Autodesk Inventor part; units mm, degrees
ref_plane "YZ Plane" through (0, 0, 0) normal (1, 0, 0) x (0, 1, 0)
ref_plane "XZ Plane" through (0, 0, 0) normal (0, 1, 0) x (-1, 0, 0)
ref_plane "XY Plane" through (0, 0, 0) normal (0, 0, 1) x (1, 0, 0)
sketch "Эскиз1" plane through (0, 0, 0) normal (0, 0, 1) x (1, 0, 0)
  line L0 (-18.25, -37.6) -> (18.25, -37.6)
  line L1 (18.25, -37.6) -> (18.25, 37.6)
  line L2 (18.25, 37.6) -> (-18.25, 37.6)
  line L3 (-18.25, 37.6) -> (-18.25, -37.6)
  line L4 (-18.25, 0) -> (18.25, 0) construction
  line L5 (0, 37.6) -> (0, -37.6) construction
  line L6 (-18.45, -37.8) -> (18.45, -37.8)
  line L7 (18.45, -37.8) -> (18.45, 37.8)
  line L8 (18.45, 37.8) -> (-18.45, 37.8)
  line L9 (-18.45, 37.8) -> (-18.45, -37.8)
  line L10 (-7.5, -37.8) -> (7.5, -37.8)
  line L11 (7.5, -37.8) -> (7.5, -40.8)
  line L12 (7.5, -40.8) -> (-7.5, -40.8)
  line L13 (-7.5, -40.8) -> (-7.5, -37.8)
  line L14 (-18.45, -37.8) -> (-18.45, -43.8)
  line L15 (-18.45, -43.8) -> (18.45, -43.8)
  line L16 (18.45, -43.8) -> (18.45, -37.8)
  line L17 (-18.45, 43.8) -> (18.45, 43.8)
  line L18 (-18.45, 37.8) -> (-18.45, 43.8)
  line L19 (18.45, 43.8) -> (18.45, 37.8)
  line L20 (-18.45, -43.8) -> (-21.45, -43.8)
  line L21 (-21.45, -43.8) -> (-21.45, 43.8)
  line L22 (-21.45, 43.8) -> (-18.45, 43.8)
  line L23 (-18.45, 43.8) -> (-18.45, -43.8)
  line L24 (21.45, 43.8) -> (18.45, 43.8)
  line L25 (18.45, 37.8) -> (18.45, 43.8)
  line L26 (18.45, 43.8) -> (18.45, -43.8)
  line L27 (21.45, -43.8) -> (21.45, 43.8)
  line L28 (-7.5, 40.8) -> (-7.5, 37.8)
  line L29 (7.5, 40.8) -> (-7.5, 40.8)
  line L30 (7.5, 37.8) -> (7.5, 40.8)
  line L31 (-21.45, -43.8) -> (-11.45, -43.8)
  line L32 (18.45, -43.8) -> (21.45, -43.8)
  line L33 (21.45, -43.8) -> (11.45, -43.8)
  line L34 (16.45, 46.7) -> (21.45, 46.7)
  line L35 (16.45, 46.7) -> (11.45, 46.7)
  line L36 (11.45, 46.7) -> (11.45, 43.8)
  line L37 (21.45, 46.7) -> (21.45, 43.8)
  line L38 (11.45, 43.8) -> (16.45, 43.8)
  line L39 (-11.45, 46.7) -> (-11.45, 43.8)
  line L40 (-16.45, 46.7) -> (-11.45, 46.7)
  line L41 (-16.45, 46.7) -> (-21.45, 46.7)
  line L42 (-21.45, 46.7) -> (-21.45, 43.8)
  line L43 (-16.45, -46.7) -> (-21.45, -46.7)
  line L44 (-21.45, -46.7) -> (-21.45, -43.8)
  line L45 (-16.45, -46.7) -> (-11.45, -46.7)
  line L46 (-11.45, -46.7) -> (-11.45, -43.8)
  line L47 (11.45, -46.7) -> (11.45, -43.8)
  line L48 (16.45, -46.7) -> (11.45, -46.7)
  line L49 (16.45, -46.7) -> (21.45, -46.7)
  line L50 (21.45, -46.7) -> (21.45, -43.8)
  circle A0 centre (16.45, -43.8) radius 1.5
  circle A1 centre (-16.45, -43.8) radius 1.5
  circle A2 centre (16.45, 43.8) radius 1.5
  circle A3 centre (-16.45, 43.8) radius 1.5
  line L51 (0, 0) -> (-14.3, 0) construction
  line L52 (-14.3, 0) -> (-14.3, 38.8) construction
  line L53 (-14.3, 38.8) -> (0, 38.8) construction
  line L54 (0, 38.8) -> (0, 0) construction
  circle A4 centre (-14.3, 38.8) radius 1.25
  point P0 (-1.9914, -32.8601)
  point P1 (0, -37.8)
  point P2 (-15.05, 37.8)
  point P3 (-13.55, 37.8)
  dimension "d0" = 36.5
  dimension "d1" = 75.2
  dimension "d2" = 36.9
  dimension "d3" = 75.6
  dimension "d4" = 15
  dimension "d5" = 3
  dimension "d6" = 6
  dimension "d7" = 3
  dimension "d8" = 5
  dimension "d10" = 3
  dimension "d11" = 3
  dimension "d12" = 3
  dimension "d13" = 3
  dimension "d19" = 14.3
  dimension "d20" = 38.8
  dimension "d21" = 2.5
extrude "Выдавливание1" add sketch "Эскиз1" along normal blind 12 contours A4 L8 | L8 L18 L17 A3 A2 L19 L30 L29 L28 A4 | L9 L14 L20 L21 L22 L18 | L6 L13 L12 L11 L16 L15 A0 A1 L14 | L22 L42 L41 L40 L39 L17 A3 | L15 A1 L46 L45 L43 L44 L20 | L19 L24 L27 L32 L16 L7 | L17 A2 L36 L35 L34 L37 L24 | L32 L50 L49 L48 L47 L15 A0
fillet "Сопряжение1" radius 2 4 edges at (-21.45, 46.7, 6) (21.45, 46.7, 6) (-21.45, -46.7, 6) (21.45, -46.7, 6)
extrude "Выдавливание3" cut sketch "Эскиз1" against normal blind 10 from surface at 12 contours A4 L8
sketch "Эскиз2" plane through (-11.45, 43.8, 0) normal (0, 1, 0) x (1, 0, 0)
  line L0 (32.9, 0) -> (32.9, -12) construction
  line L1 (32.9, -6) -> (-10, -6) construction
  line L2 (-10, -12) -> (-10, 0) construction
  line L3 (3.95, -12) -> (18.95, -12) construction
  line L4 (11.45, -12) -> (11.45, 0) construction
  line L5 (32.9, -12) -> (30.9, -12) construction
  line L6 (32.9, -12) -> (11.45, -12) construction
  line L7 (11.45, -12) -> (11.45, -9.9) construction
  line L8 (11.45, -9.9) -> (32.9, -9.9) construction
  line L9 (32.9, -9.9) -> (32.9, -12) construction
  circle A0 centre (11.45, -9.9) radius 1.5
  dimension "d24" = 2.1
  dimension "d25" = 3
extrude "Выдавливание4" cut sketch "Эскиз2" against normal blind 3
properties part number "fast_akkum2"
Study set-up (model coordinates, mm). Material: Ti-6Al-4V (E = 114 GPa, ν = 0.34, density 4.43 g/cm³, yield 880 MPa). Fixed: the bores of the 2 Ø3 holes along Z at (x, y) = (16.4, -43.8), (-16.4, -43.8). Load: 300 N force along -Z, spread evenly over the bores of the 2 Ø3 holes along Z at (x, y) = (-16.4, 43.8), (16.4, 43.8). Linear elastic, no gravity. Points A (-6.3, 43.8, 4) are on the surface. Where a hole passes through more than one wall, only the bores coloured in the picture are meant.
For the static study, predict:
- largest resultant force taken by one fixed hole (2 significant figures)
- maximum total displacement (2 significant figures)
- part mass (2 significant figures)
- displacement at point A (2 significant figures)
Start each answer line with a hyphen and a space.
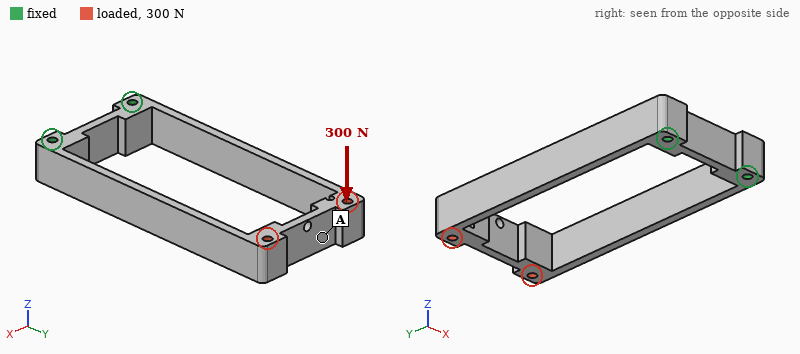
- 150 N
- 0.71 mm
- 51 g
- 0.67 mm
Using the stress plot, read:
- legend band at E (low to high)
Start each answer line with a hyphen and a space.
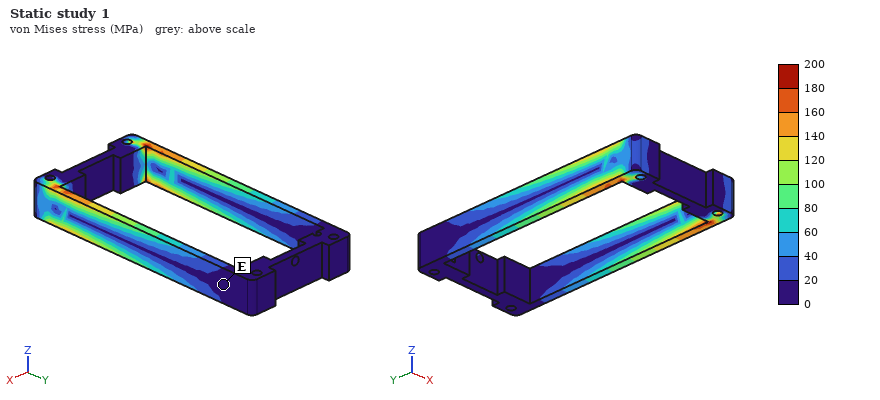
- 0 to 20 MPa
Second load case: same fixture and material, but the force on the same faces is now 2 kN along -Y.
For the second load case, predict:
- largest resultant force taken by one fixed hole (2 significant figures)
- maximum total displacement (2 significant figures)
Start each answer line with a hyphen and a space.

- 1.0 kN
- 0.14 mm
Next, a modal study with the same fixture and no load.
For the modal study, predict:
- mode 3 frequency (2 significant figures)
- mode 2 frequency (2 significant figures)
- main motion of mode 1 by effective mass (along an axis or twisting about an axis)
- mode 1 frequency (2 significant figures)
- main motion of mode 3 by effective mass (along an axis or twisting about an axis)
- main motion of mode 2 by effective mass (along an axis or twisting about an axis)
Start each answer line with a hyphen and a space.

- 1400 Hz
- 810 Hz
- along X
- 410 Hz
- twisting about Y
- along Z
